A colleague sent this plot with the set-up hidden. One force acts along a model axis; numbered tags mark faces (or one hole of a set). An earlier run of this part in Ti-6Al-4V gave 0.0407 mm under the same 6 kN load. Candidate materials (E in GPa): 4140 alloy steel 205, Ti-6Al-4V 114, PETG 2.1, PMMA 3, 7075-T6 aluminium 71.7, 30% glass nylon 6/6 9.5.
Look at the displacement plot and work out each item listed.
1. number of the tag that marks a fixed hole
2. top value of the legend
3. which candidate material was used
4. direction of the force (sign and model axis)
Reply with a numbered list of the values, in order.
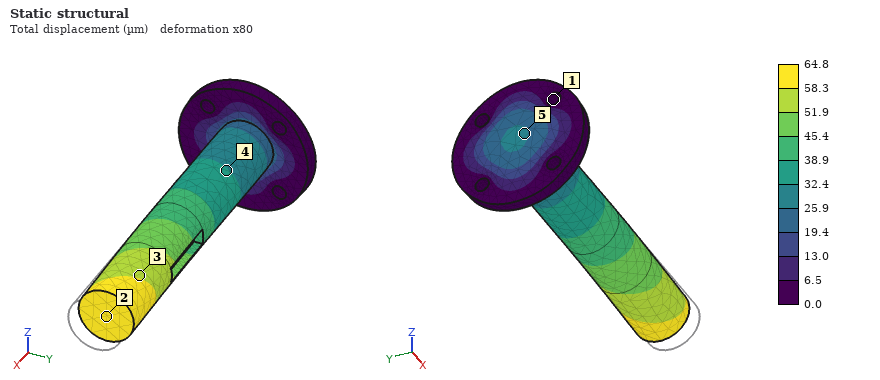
1. 1
2. 64.8 µm
3. 7075-T6 aluminium
4. -X
